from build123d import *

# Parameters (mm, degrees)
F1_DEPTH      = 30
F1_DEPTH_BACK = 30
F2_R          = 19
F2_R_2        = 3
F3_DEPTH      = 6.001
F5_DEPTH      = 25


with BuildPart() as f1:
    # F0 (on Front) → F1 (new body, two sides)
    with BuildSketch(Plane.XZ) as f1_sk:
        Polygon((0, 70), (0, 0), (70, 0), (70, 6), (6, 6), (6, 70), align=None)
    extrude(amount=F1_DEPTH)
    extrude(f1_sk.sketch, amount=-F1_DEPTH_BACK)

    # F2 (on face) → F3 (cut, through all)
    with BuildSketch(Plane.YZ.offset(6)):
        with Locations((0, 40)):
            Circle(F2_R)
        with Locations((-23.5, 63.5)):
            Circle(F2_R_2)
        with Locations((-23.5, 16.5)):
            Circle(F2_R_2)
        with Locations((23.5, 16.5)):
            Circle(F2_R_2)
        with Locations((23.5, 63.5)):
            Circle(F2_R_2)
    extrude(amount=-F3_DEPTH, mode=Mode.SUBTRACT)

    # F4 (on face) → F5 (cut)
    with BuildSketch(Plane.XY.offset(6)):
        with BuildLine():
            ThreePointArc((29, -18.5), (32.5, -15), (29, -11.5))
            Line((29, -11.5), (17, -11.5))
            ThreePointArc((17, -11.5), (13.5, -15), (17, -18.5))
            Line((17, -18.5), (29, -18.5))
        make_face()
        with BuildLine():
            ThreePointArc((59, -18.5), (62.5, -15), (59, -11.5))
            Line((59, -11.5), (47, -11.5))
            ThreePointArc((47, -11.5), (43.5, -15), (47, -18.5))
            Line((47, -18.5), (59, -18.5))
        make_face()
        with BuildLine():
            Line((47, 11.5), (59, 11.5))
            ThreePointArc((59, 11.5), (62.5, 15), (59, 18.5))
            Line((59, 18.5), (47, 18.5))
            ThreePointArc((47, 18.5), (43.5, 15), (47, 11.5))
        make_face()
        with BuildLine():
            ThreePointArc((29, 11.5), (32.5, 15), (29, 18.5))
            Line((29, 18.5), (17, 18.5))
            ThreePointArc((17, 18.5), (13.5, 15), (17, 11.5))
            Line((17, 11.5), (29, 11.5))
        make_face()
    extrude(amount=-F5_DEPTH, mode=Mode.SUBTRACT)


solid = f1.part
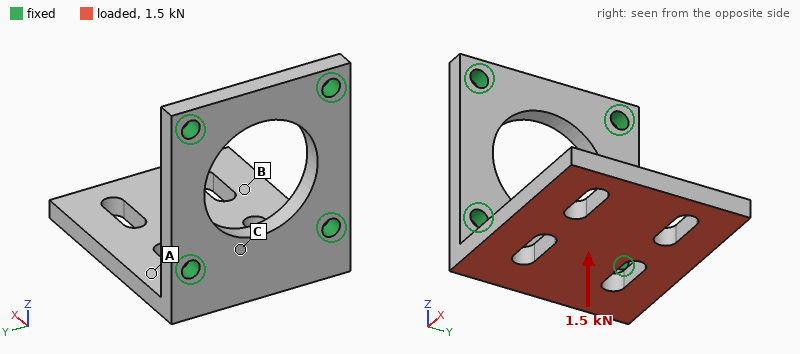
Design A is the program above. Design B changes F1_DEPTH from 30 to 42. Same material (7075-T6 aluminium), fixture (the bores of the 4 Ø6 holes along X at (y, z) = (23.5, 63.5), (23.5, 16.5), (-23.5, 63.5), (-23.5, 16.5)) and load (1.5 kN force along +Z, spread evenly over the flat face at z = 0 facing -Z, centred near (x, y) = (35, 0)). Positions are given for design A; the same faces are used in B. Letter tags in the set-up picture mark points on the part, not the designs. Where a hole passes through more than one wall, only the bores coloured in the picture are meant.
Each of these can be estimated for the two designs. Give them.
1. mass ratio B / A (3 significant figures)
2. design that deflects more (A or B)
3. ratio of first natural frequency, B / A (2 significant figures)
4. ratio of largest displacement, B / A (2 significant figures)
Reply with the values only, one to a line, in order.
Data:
1.26
A
1.00
0.82
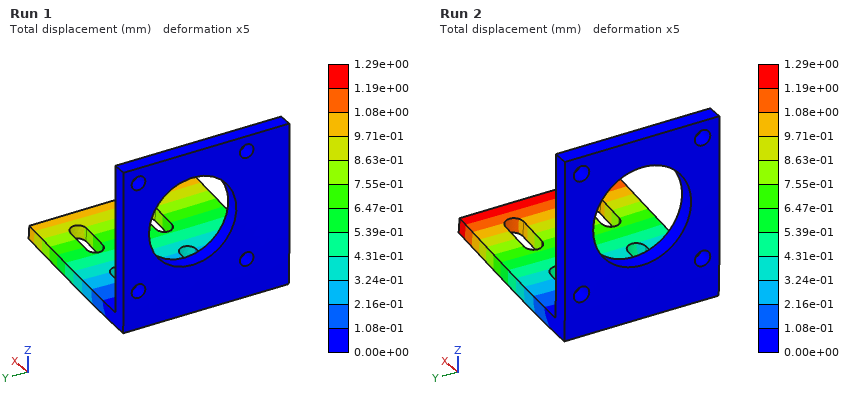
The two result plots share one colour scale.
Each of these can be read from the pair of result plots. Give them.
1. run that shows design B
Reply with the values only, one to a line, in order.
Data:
Run 1
